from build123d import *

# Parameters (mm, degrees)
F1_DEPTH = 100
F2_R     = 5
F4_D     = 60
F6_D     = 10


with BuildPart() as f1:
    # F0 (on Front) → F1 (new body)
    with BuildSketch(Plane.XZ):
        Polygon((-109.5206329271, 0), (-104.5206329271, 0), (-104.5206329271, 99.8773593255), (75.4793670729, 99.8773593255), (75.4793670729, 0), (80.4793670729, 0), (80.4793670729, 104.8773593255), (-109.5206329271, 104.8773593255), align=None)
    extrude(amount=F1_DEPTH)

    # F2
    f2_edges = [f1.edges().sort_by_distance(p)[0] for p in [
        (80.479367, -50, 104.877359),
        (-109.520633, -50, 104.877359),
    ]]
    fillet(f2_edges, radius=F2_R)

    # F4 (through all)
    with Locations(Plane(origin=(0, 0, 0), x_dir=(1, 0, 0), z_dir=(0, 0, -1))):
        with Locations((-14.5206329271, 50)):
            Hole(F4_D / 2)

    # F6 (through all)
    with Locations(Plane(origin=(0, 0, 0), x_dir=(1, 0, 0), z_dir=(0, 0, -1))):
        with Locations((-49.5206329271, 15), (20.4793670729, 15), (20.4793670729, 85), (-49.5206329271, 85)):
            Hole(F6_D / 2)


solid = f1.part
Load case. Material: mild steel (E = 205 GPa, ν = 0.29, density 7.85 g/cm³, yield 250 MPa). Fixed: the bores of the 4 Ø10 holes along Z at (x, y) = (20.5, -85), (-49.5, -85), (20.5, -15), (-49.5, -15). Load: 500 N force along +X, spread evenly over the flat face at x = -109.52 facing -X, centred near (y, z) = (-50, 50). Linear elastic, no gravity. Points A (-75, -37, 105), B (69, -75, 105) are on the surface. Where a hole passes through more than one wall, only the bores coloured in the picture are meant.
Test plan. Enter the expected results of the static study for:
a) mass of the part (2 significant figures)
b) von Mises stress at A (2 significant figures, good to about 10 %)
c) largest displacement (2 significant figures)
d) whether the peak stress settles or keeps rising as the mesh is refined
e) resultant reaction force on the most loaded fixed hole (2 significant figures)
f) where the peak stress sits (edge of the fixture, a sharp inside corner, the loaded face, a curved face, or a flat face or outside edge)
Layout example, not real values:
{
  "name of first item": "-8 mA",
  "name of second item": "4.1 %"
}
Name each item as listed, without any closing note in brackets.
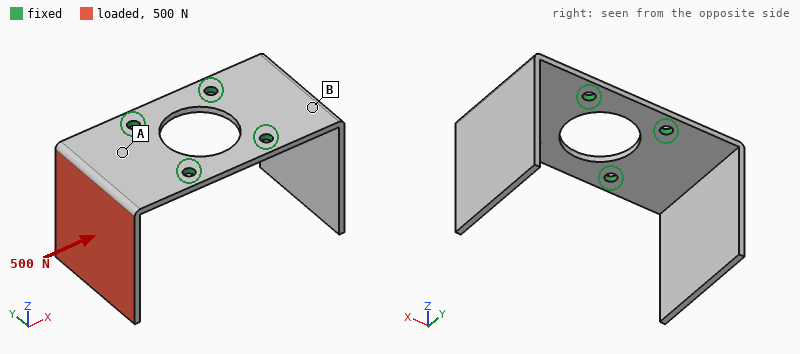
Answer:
{
  "mass of the part": "1.4 kg",
  "von Mises stress at A": "53 MPa",
  "largest displacement": "1.0 mm",
  "whether the peak stress settles or keeps rising as the mesh is refined": "keeps rising",
  "resultant reaction force on the most loaded fixed hole": "260 N",
  "where the peak stress sits": "edge of the fixture"
}
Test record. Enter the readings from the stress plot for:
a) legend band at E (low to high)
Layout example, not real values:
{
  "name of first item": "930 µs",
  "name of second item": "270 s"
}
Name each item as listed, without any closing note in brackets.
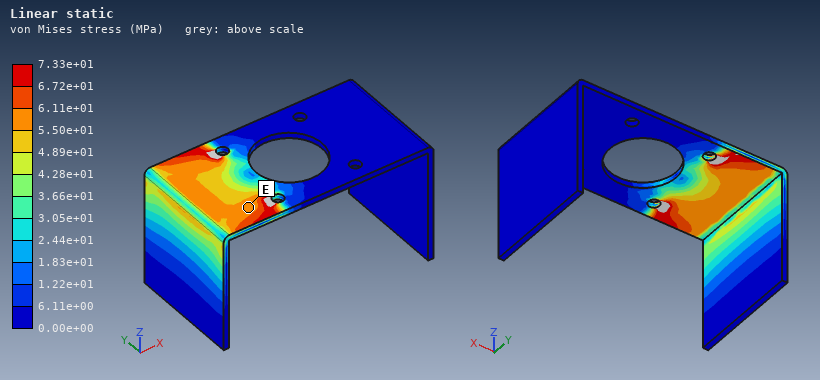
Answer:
{
  "legend band at E": "5.50e+01 to 6.11e+01 MPa"
}
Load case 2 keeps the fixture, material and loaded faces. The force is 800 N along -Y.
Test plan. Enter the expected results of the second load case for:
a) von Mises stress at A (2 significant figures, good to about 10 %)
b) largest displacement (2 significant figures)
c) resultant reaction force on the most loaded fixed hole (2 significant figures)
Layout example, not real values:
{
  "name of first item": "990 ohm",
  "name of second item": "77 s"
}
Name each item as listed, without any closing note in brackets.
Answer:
{
  "von Mises stress at A": "43 MPa",
  "largest displacement": "0.36 mm",
  "resultant reaction force on the most loaded fixed hole": "910 N"
}
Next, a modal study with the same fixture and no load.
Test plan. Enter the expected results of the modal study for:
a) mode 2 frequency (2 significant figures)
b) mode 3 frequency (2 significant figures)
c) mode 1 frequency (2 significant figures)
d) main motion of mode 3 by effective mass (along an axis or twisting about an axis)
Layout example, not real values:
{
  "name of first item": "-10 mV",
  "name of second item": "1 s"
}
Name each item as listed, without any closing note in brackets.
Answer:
{
  "mode 2 frequency": "210 Hz",
  "mode 3 frequency": "430 Hz",
  "mode 1 frequency": "210 Hz",
  "main motion of mode 3 by effective mass": "along Y"
}
